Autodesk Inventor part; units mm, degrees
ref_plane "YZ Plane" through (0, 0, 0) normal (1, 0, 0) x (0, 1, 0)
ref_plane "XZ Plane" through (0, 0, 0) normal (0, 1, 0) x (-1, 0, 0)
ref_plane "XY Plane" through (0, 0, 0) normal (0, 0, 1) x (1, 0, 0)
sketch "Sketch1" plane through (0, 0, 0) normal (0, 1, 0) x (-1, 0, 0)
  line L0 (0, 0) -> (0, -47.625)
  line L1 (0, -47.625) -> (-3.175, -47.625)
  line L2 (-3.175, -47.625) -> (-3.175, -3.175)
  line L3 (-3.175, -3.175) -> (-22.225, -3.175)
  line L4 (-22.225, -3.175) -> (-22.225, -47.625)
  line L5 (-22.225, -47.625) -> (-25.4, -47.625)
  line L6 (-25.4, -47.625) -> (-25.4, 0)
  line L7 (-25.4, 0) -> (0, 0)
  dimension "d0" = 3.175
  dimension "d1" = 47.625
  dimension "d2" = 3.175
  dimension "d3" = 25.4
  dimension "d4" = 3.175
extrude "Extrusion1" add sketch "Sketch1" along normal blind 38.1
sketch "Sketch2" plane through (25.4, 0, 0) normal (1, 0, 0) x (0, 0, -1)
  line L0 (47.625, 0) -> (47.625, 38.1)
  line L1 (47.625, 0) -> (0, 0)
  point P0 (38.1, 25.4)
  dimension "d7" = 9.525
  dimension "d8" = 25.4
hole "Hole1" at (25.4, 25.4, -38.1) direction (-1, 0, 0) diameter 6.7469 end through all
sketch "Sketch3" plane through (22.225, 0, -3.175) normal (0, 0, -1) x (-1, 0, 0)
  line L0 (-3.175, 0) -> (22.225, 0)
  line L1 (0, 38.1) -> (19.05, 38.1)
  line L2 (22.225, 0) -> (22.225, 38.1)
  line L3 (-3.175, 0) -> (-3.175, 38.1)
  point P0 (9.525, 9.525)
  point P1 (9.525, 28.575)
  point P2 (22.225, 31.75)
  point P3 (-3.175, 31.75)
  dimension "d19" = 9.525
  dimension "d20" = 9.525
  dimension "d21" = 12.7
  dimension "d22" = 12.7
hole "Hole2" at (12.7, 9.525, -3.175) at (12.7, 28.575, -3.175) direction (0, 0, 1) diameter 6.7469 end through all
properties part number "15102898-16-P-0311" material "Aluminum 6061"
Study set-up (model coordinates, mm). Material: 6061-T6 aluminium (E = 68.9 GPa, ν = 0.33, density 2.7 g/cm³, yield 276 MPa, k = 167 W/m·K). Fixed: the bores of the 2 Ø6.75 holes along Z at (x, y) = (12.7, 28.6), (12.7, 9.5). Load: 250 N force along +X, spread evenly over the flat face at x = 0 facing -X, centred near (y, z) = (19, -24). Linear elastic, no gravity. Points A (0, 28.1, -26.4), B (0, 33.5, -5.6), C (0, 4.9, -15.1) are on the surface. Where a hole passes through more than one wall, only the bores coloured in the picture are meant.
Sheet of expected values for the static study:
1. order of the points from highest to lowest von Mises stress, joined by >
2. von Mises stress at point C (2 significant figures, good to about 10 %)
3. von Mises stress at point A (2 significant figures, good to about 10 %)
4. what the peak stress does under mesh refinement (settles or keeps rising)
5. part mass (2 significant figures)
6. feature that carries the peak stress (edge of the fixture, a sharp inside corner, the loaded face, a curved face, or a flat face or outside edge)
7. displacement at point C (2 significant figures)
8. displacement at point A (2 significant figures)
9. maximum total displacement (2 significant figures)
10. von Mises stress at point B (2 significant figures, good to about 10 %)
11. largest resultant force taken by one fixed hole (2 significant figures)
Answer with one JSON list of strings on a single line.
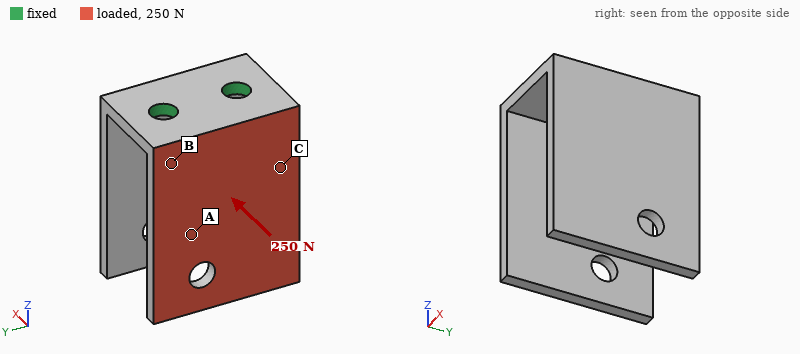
["B > C > A", "42 MPa", "17 MPa", "keeps rising", "36 g", "edge of the fixture", "0.14 mm", "0.30 mm", "0.66 mm", "63 MPa", "130 N"]
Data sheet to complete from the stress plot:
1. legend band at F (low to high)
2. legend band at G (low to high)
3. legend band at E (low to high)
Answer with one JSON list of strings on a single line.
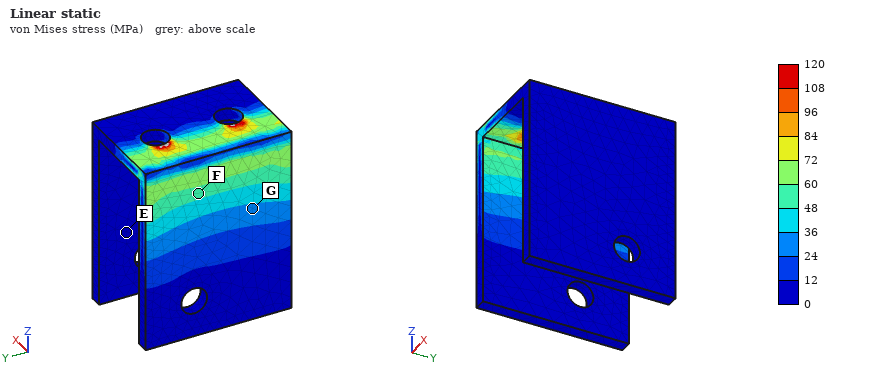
["48 to 60 MPa", "24 to 36 MPa", "0 to 12 MPa"]
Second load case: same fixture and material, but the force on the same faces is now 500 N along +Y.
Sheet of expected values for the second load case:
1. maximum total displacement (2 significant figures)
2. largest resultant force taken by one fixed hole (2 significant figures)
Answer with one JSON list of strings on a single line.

["0.11 mm", "570 N"]
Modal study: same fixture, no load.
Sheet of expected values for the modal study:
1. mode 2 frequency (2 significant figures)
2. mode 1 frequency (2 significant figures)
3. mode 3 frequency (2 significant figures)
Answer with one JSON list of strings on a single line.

["990 Hz", "990 Hz", "2700 Hz"]
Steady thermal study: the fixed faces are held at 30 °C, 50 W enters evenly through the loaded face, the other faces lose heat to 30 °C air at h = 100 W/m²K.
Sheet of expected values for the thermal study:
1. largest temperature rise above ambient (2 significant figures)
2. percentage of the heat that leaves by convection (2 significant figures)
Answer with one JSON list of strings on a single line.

["58 K", "22 %"]
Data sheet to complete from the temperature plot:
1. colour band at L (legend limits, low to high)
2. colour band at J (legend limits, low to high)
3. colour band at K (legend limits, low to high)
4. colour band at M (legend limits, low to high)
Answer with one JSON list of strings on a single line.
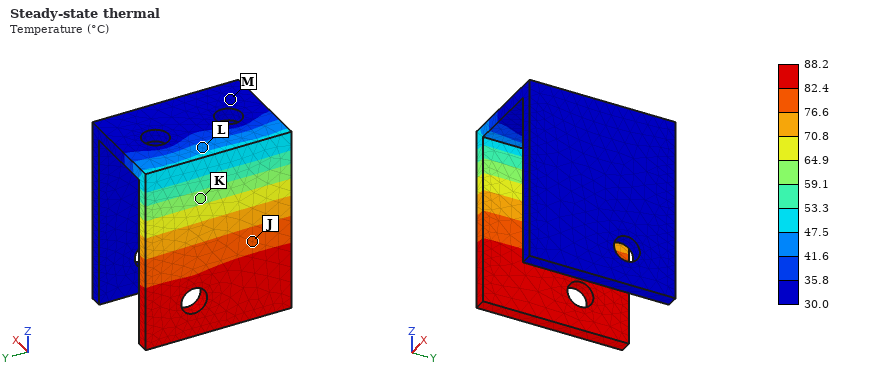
["41.6 to 47.5 °C", "76.6 to 82.4 °C", "59.1 to 64.9 °C", "30.0 to 35.8 °C"]
